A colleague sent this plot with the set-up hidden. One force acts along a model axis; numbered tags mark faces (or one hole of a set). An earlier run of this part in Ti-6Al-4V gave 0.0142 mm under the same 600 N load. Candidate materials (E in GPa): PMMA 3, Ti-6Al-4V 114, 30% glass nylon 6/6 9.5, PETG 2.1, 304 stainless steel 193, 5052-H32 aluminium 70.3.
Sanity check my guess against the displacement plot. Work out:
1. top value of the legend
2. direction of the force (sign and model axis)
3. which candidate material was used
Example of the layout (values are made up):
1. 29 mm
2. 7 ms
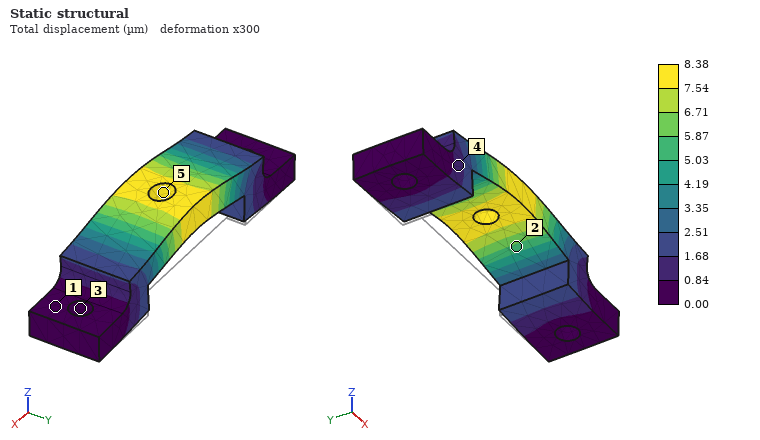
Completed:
1. 8.38 µm
2. +Z
3. 304 stainless steel
